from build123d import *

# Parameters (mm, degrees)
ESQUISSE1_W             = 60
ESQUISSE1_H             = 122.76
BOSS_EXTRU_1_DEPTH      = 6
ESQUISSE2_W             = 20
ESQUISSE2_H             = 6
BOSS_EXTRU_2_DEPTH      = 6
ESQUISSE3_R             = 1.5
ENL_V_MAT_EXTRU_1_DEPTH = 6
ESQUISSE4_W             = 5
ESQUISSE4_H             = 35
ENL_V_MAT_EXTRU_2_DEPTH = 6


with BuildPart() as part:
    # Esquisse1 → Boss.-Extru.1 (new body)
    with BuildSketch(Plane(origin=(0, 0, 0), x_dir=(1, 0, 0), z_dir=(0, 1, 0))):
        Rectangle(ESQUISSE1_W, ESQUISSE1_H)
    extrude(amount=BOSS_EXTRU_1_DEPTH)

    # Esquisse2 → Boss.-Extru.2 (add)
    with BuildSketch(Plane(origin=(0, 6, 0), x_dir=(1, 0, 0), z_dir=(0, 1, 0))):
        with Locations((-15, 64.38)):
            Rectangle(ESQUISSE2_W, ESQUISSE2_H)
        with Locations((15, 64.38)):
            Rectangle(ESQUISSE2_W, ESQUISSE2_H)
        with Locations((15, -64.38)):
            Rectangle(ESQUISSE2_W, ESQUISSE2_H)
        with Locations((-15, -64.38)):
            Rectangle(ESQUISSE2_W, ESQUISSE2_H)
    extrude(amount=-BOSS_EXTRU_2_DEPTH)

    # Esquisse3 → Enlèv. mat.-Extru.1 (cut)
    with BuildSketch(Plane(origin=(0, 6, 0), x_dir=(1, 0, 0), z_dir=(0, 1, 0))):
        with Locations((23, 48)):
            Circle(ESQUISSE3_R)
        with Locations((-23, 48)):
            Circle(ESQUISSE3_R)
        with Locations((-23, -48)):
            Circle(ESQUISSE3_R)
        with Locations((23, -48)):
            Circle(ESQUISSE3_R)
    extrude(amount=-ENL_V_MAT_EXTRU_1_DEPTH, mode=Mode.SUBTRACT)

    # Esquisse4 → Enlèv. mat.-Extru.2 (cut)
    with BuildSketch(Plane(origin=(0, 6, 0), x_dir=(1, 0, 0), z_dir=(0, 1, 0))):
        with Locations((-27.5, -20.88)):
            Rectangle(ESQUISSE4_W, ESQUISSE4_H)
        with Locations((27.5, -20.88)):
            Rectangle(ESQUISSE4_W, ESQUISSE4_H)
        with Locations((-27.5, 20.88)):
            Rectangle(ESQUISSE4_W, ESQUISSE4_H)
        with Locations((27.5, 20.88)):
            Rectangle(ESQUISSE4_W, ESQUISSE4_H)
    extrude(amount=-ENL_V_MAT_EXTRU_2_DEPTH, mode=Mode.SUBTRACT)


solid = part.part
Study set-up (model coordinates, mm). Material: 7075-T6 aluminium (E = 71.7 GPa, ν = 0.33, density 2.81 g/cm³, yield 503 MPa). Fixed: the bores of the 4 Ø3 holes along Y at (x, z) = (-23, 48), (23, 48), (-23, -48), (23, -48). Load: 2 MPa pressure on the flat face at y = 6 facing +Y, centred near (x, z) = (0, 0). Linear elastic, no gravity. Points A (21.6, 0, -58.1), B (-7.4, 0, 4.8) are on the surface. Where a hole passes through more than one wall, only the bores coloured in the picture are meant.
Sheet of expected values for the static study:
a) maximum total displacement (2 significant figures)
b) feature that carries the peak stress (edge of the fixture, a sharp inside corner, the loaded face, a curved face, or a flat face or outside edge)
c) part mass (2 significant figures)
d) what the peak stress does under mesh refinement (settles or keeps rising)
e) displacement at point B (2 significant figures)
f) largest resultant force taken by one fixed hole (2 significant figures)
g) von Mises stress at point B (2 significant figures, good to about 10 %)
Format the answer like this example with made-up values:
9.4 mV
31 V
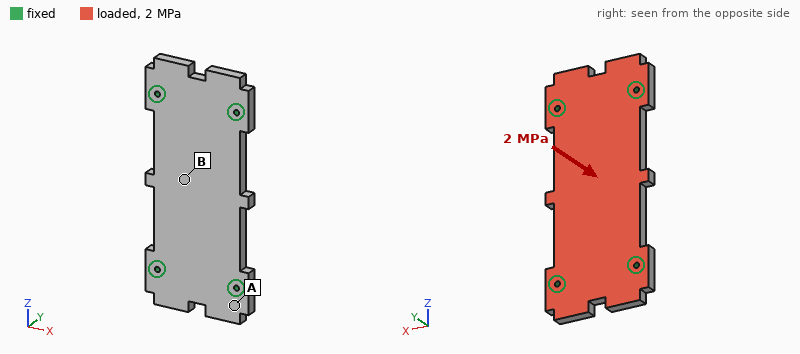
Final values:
0.50 mm
edge of the fixture
120 g
keeps rising
0.45 mm
3.6 kN
130 MPa
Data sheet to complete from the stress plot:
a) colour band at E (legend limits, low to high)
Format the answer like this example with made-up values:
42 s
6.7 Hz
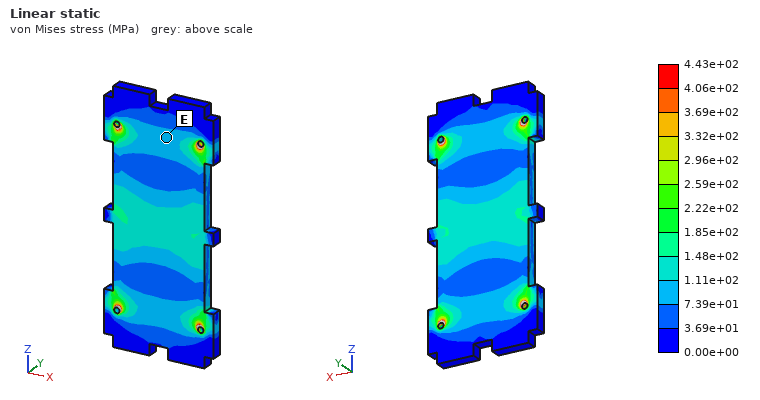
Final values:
7.39e+01 to 1.11e+02 MPa
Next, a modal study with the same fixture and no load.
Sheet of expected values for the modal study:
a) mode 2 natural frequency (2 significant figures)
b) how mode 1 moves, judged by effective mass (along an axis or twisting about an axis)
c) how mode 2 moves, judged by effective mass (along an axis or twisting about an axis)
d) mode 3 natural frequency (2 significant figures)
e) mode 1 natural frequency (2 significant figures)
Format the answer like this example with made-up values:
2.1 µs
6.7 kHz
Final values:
4900 Hz
along Y
twisting about Z
7400 Hz
2800 Hz
